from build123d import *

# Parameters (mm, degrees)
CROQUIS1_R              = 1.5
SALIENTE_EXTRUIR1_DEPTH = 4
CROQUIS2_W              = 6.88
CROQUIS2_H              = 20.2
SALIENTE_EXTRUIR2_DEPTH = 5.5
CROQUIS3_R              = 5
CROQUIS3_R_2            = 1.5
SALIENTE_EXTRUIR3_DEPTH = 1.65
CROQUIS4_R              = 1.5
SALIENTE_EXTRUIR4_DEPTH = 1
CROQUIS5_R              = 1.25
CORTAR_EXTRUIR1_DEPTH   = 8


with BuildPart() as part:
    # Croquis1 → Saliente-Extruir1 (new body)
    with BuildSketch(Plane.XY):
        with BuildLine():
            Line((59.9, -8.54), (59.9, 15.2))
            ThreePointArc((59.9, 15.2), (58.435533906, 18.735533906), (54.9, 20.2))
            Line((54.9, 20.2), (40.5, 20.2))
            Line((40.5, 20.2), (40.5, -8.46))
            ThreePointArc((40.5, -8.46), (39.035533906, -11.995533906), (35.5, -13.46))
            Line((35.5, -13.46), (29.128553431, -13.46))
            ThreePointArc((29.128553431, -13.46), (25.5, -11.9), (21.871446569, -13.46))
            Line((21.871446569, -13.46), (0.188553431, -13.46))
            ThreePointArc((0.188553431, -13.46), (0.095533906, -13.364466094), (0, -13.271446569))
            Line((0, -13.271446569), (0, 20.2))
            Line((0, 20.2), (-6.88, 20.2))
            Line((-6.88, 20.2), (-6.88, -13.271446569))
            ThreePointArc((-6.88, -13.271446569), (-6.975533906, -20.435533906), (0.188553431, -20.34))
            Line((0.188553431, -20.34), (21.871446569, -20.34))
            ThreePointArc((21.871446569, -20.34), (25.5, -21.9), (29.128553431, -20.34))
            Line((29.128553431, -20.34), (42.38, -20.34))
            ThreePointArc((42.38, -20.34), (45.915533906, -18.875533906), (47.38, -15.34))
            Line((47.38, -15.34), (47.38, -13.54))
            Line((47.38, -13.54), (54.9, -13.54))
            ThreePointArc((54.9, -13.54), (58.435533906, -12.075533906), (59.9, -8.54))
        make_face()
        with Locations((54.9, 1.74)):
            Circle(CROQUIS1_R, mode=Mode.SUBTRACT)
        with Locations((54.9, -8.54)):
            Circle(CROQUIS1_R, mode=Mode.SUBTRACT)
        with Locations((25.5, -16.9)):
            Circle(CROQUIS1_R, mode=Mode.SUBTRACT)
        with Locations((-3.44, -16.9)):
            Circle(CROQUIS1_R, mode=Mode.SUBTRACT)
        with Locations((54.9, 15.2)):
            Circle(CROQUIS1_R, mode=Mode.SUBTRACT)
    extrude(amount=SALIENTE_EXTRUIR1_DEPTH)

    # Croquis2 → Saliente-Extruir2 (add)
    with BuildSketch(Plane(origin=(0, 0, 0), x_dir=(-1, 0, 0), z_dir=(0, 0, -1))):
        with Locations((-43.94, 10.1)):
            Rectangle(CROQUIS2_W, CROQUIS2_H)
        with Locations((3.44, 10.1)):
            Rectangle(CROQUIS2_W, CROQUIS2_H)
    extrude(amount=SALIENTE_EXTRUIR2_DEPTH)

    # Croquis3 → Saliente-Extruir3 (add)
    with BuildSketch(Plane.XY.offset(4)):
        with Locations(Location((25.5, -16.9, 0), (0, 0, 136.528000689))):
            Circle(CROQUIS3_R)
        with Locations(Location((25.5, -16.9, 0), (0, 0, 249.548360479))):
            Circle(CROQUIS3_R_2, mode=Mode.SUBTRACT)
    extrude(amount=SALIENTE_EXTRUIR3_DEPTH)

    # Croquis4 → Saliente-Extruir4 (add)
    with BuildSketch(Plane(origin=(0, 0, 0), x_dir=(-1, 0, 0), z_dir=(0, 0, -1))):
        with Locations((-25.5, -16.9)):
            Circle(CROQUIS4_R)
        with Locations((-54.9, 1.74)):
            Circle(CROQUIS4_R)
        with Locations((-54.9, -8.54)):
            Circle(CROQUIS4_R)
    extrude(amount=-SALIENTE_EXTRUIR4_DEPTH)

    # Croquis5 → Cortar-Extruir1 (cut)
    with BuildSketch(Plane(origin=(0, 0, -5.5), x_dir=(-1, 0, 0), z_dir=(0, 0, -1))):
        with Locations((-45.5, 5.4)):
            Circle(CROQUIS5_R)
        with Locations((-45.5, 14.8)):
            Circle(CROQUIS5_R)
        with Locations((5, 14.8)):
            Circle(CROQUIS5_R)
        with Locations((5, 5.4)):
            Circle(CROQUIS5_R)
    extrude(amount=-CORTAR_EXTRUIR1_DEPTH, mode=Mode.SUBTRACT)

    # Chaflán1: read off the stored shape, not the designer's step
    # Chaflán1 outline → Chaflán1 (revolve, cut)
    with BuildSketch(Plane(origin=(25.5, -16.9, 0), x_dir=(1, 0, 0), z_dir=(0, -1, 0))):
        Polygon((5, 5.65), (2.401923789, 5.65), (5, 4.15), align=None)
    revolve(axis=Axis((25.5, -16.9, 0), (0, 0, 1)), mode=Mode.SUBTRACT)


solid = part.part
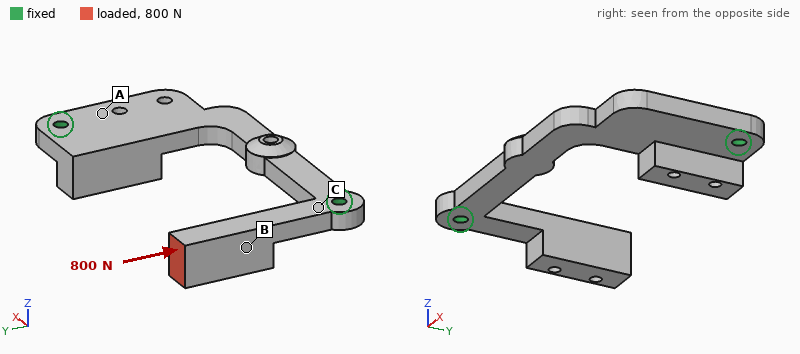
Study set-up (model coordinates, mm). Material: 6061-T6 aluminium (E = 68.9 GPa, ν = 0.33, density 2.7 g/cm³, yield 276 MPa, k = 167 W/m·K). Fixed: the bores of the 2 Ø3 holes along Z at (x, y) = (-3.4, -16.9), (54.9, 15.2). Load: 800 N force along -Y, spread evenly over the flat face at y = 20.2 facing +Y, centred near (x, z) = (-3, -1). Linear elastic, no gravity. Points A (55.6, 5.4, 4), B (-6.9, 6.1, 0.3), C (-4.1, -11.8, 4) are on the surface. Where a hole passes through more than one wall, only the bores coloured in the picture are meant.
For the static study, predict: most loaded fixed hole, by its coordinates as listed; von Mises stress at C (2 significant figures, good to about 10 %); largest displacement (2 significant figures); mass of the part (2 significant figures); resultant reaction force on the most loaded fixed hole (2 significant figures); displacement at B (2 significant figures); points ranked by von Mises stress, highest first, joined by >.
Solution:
(-3.4, -16.9)
85 MPa
0.43 mm
17 g
800 N
0.20 mm
C > B > A
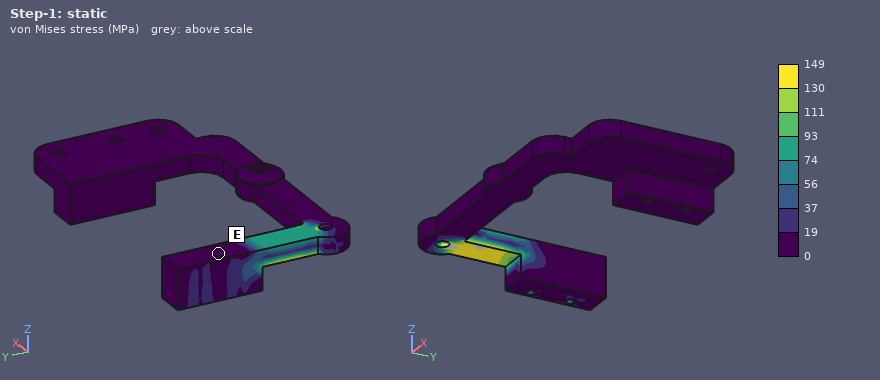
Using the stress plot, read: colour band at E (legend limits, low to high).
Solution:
0 to 19 MPa
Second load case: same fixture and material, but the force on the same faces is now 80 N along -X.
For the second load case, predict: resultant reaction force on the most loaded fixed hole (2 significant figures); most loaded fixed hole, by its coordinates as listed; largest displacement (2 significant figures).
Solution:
93 N
(-3.4, -16.9)
0.19 mm
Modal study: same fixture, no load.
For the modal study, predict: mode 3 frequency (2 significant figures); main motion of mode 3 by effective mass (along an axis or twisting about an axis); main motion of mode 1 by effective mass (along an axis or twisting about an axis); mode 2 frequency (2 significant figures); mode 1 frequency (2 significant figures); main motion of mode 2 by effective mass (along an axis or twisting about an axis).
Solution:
3000 Hz
along Z
along Z
2700 Hz
1700 Hz
along X
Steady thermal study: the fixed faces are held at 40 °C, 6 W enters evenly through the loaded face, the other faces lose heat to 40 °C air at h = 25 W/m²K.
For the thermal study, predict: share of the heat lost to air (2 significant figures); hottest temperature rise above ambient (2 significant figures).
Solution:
11 %
32 K
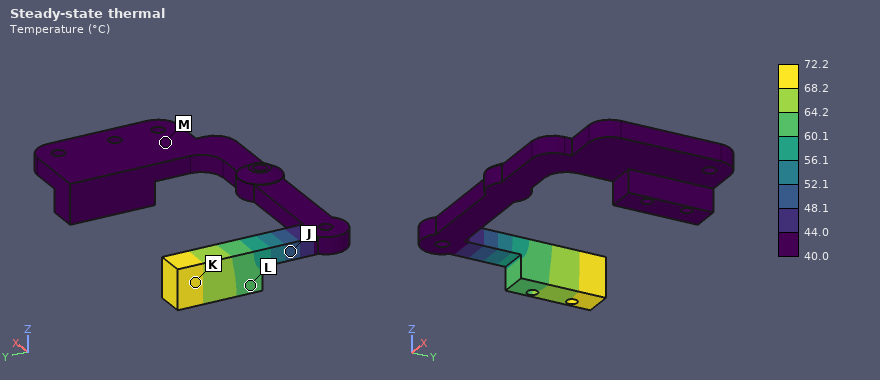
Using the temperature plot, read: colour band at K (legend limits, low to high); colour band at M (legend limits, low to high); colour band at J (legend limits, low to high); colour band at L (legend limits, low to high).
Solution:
68.2 to 72.2 °C
40.0 to 44.0 °C
48.1 to 52.1 °C
60.1 to 64.2 °C
